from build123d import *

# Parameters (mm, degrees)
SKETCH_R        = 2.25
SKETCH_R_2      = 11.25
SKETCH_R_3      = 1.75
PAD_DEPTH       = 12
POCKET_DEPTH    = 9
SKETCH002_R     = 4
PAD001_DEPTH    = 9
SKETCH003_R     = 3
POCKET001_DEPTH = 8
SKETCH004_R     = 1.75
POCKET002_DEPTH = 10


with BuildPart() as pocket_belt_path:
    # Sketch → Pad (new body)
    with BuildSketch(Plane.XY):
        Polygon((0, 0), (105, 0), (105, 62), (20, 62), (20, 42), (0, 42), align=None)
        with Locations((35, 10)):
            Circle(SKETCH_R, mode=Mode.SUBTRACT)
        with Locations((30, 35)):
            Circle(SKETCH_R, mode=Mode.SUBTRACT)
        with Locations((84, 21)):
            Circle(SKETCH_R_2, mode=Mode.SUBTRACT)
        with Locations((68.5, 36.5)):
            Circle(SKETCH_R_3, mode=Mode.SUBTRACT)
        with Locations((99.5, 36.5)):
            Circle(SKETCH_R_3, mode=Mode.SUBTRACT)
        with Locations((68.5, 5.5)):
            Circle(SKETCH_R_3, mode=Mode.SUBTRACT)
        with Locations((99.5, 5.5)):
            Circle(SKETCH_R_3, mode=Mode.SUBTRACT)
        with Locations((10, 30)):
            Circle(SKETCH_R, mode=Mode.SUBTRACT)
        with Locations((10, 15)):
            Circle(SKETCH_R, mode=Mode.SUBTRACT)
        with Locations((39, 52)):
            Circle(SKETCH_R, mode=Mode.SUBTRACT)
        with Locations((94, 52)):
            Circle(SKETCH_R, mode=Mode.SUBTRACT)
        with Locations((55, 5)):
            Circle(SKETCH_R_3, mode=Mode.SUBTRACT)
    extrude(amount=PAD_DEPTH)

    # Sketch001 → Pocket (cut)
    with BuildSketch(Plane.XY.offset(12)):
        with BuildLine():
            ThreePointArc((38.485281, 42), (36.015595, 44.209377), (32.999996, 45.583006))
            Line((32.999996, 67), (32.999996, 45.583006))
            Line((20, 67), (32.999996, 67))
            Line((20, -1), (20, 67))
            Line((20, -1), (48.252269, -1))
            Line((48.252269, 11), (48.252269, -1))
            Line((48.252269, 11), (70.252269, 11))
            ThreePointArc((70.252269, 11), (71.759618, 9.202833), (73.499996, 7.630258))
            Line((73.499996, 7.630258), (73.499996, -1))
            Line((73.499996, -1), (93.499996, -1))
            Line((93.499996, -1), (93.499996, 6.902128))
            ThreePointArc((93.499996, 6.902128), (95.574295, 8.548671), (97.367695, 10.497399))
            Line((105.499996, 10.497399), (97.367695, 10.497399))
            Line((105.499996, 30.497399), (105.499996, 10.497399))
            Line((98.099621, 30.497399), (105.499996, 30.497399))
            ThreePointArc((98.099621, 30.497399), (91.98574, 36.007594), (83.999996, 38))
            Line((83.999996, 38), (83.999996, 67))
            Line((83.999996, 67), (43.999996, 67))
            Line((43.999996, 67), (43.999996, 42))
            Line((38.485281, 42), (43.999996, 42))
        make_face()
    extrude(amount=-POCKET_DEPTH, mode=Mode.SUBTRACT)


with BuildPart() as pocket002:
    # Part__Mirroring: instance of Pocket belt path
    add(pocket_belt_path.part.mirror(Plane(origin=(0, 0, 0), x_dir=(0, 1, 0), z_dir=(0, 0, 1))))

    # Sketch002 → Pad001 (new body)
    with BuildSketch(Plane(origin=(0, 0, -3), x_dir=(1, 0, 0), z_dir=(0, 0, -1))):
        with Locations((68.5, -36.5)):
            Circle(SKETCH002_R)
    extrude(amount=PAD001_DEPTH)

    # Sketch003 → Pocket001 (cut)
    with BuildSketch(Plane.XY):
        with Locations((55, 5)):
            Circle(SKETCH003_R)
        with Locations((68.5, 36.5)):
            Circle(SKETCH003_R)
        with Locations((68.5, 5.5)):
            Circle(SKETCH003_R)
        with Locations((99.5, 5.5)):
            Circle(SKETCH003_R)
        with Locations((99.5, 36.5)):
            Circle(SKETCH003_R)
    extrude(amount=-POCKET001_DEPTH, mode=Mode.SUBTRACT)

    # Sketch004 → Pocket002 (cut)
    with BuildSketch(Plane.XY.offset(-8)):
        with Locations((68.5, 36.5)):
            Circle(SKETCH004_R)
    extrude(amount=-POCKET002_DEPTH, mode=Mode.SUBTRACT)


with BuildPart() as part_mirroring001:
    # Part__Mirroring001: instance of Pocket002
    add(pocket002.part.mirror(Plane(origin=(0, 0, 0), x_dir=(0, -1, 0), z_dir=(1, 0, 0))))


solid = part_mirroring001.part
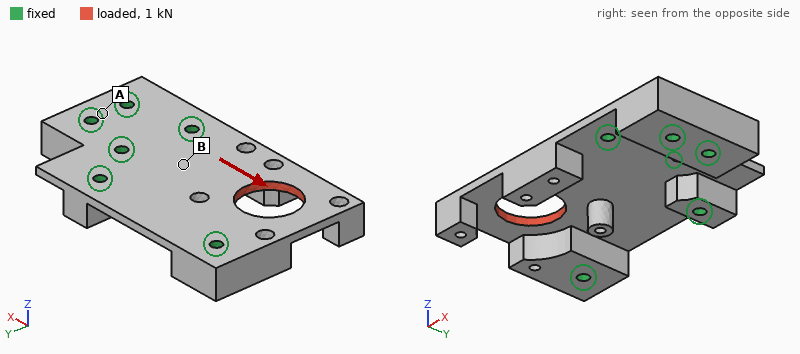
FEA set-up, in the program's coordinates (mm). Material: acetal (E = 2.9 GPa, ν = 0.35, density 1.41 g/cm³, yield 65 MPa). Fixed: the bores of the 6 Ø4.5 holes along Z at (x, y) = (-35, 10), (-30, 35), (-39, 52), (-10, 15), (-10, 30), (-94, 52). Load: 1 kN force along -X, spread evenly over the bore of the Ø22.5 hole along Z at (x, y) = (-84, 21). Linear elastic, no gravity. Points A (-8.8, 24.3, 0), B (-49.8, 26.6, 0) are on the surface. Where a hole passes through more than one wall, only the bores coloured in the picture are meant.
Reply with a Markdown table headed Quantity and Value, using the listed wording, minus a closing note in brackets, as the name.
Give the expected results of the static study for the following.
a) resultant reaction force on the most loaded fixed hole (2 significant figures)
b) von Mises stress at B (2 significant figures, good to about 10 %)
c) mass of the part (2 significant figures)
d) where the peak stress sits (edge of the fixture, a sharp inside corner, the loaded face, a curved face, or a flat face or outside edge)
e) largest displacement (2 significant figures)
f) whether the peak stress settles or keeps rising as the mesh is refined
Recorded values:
| Quantity | Value |
|---|---|
| resultant reaction force on the most loaded fixed hole | 350 N |
| von Mises stress at B | 3.3 MPa |
| mass of the part | 47 g |
| where the peak stress sits | a sharp inside corner |
| largest displacement | 0.22 mm |
| whether the peak stress settles or keeps rising as the mesh is refined | keeps rising |
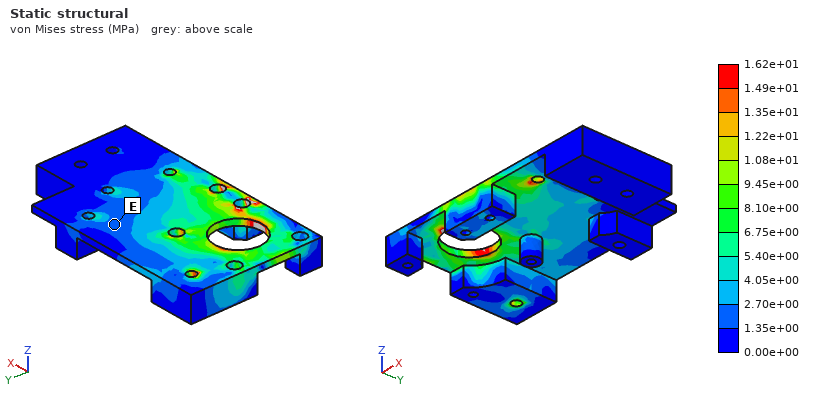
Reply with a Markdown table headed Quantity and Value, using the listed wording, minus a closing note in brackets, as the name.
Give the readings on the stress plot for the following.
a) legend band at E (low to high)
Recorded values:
| Quantity | Value |
|---|---|
| legend band at E | 1.35e+00 to 2.70e+00 MPa |
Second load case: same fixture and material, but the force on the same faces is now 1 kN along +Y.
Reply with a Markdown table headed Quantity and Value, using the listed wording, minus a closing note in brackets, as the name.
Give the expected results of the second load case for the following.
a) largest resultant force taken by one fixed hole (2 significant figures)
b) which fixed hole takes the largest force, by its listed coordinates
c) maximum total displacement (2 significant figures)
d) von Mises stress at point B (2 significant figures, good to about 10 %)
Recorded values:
| Quantity | Value |
|---|---|
| largest resultant force taken by one fixed hole | 710 N |
| which fixed hole takes the largest force, by its listed coordinates | (-94, 52) |
| maximum total displacement | 0.30 mm |
| von Mises stress at point B | 4.4 MPa |
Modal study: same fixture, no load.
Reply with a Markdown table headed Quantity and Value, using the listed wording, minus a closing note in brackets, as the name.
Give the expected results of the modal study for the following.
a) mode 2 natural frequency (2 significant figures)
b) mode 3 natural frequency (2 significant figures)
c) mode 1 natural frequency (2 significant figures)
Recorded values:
| Quantity | Value |
|---|---|
| mode 2 natural frequency | 930 Hz |
| mode 3 natural frequency | 1700 Hz |
| mode 1 natural frequency | 460 Hz |
